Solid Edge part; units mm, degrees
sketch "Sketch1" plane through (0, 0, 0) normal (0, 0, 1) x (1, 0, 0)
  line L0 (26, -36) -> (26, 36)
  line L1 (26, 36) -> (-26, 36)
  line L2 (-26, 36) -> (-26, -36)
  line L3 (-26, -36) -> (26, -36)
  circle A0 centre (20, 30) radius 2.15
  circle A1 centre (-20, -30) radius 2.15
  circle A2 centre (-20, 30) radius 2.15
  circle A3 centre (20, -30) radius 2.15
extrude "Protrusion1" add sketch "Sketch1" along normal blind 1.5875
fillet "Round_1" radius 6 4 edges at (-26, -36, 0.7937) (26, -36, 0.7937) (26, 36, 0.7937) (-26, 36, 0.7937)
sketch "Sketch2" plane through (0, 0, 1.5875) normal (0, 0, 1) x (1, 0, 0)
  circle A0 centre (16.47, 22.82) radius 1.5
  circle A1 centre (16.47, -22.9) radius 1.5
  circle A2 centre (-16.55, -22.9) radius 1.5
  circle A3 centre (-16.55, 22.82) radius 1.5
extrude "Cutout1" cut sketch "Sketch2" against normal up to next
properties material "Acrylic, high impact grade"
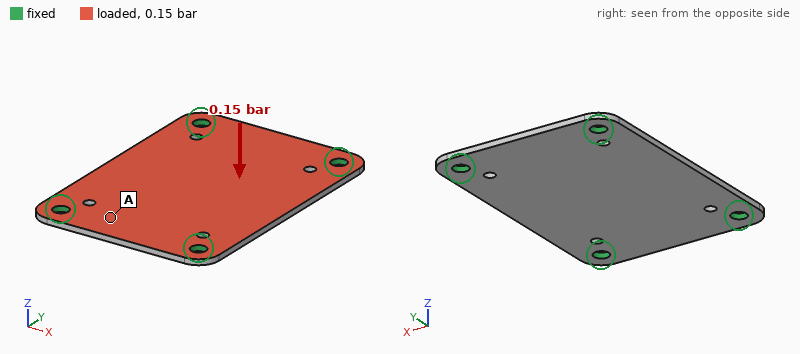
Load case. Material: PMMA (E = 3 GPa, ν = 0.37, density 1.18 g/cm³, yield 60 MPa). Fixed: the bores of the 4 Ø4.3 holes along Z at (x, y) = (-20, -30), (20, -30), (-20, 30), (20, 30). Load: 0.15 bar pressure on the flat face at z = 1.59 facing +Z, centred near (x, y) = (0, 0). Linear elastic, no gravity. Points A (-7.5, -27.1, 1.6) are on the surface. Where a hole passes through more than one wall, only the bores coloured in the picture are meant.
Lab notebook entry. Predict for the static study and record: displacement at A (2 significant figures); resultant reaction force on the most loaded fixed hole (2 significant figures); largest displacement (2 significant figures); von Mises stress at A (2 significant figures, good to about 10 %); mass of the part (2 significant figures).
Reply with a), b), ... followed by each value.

a) 0.13 mm
b) 14 N
c) 0.60 mm
d) 3.3 MPa
e) 6.8 g
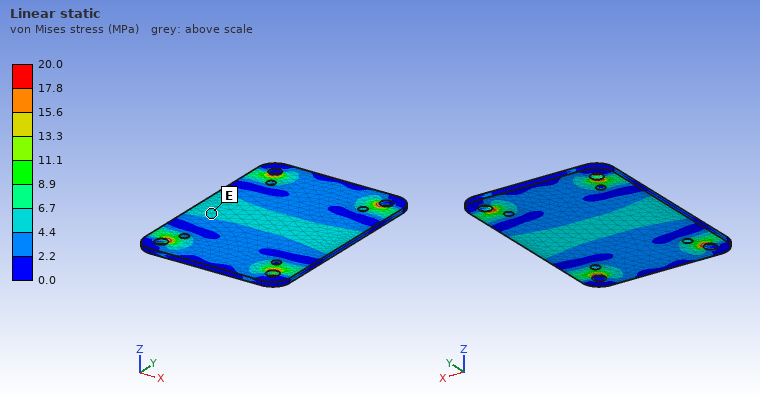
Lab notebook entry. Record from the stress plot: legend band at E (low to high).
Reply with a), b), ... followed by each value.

a) 4.4 to 6.7 MPa
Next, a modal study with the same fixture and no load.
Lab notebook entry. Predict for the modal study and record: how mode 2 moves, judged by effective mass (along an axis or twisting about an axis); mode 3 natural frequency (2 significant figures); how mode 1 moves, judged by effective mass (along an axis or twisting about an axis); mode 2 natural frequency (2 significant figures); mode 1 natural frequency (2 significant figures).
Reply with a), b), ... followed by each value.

a) twisting about Y
b) 1500 Hz
c) along Z
d) 960 Hz
e) 680 Hz
